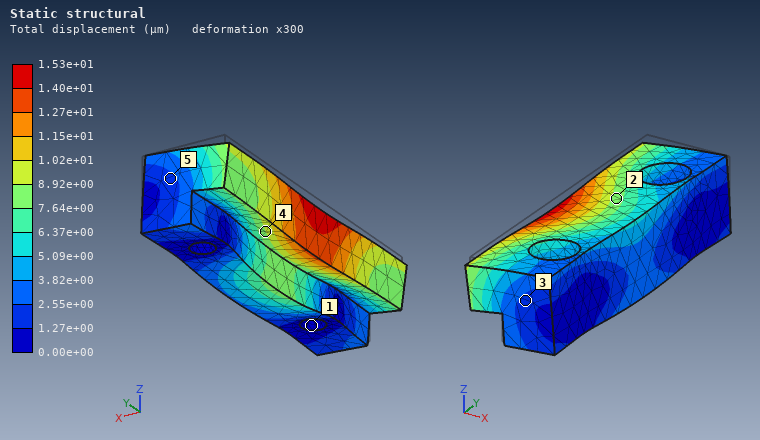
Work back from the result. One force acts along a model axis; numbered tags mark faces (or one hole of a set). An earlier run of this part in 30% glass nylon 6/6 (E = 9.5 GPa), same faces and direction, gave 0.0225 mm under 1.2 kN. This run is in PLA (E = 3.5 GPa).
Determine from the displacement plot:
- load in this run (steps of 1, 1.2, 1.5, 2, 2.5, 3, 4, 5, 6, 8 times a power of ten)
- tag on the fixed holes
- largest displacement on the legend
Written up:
300 N
1
1.53e+01 µm
